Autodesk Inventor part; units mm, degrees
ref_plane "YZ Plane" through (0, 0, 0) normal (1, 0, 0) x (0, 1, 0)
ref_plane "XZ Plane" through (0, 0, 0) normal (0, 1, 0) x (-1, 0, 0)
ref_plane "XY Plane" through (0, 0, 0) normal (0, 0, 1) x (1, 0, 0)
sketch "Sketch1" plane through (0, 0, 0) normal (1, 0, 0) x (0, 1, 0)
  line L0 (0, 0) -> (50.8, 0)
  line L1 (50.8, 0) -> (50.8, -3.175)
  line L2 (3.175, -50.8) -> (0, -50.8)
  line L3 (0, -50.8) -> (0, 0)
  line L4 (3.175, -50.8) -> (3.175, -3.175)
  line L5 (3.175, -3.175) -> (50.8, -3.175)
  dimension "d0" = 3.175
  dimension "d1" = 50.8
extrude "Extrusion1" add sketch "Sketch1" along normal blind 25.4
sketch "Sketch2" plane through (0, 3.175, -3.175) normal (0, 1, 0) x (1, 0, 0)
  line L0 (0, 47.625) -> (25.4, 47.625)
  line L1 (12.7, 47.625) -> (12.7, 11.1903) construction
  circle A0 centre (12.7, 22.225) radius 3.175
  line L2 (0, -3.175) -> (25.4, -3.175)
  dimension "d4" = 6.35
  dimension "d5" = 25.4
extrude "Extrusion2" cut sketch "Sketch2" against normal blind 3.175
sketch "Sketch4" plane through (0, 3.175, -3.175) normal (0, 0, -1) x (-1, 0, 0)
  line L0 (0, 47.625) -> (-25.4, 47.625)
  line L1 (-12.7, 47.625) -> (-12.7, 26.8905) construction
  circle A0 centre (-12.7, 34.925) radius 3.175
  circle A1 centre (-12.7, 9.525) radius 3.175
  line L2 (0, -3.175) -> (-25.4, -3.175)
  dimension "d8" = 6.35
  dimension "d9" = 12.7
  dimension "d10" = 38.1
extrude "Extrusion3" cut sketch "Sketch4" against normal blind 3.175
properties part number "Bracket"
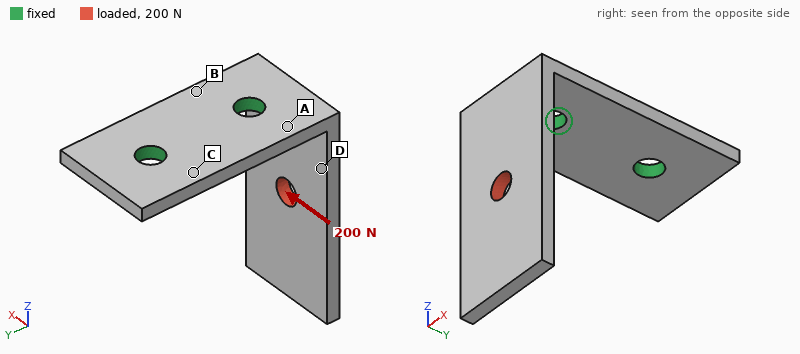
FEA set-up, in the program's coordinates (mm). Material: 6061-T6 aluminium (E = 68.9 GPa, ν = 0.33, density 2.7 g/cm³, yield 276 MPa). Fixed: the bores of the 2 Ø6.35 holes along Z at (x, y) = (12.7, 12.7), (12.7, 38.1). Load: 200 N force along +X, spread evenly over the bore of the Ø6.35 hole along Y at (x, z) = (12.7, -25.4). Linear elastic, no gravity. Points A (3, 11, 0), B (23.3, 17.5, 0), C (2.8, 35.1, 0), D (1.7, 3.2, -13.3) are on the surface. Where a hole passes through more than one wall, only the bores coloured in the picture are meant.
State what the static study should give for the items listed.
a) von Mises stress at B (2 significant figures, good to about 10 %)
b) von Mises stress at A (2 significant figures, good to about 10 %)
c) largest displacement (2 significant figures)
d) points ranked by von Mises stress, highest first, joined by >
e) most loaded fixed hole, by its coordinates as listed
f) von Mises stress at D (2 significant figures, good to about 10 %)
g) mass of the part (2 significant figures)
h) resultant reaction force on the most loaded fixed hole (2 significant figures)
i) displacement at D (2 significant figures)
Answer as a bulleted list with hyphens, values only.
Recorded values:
- 32 MPa
- 45 MPa
- 0.25 mm
- A > B > D > C
- (12.7, 12.7)
- 16 MPa
- 21 g
- 250 N
- 0.079 mm
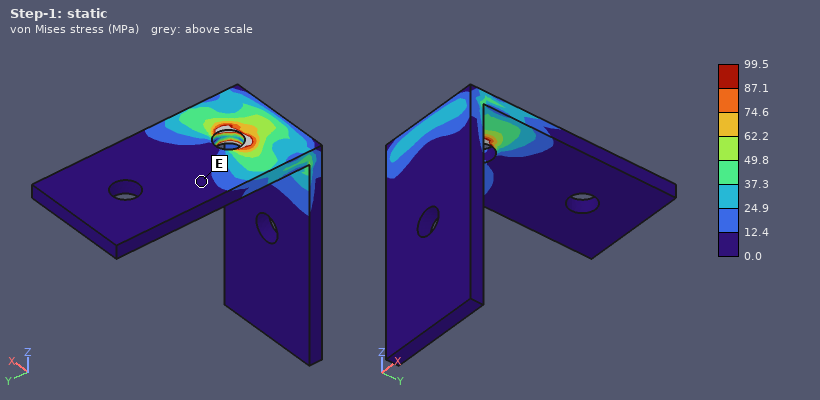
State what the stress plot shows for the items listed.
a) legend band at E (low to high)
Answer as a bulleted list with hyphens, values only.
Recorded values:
- 0.0 to 12.4 MPa
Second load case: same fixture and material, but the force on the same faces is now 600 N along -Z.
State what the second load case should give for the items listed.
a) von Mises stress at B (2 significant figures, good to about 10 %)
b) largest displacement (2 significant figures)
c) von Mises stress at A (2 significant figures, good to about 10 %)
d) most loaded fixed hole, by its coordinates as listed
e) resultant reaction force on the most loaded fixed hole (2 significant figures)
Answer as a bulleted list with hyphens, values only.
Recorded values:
- 17 MPa
- 0.31 mm
- 49 MPa
- (12.7, 12.7)
- 630 N
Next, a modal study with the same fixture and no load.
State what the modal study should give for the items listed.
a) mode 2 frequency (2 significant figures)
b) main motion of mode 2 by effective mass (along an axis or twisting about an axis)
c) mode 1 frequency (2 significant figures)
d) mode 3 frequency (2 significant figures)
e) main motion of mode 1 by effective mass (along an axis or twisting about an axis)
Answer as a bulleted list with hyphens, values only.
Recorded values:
- 1600 Hz
- along X
- 830 Hz
- 4000 Hz
- along Y
